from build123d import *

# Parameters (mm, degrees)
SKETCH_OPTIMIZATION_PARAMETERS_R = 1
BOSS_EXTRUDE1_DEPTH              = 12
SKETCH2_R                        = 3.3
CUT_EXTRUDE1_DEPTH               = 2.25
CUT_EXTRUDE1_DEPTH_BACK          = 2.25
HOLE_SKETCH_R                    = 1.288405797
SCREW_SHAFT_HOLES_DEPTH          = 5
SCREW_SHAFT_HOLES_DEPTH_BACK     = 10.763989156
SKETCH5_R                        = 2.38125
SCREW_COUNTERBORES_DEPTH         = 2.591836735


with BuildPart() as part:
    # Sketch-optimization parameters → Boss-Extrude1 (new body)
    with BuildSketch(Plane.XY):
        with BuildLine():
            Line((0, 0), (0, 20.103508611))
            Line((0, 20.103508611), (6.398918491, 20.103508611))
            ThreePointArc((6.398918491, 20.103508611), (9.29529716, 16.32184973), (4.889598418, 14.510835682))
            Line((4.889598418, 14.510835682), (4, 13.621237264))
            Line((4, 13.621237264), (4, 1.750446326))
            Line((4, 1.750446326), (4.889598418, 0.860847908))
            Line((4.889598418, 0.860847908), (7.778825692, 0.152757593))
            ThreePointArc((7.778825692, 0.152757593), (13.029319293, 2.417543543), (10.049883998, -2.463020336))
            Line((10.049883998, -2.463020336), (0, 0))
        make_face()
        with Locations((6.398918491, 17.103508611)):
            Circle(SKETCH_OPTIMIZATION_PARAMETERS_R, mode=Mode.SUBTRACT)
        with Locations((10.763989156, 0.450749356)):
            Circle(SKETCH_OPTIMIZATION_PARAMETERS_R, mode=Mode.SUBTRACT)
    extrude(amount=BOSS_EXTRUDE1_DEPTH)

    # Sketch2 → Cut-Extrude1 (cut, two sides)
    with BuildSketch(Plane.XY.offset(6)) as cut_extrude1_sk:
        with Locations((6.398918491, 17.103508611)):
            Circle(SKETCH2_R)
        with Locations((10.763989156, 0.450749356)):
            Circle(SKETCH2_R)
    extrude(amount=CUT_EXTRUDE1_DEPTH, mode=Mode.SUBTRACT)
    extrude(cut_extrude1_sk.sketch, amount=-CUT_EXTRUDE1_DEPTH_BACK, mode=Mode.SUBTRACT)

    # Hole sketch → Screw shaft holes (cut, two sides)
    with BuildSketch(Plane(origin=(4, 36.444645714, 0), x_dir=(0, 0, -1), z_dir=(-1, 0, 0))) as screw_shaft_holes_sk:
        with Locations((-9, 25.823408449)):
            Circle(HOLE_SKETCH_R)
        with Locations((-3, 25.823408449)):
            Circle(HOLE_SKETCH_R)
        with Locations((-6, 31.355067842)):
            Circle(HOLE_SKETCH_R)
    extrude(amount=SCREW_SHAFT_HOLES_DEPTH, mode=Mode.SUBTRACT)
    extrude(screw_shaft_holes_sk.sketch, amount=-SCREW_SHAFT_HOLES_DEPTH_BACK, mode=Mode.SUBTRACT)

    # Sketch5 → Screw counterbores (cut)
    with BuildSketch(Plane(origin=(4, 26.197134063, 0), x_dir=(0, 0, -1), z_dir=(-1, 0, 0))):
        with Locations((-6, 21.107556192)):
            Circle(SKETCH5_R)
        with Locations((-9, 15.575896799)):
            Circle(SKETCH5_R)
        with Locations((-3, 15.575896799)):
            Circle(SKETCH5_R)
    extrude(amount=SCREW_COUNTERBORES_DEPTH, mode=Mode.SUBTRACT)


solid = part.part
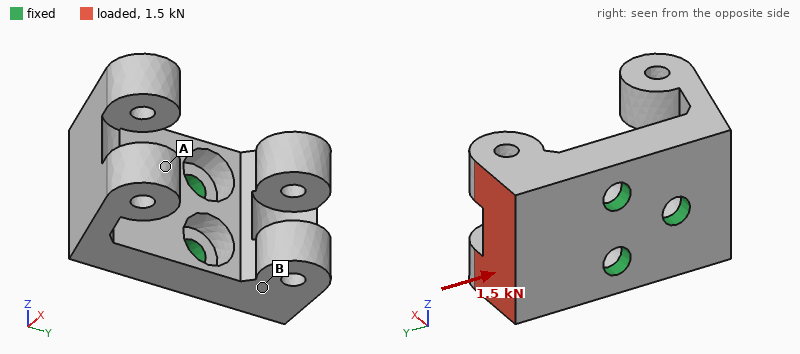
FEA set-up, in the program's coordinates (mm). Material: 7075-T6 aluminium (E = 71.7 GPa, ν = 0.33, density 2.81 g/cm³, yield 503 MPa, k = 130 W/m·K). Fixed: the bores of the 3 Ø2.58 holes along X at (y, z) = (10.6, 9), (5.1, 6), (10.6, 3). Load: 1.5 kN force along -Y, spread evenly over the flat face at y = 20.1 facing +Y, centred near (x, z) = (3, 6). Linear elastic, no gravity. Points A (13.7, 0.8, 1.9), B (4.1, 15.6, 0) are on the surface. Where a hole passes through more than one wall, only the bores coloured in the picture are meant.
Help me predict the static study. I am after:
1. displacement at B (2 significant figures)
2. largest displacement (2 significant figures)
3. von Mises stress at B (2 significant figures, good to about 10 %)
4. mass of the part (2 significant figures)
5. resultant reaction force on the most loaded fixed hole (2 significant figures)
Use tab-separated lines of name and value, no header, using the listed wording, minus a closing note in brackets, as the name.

displacement at B	32 µm
largest displacement	72 µm
von Mises stress at B	54 MPa
mass of the part	3.7 g
resultant reaction force on the most loaded fixed hole	590 N
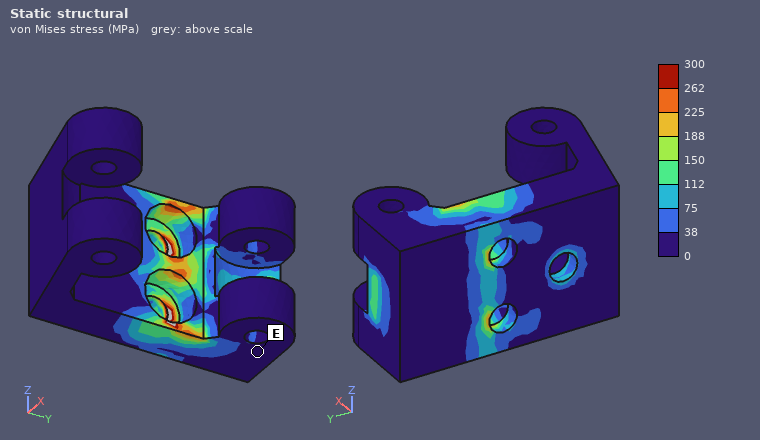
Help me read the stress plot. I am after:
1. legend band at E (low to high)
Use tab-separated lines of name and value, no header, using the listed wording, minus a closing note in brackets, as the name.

legend band at E	0 to 38 MPa
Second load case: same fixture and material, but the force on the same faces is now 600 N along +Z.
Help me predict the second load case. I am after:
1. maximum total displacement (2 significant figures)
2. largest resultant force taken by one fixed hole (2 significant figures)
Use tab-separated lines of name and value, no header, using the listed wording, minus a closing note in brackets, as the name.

maximum total displacement	21 µm
largest resultant force taken by one fixed hole	730 N
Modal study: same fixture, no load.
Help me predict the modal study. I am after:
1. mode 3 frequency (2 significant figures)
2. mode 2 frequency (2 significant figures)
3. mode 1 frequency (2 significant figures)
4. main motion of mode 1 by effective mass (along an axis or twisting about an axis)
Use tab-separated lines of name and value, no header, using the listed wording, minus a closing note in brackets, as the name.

mode 3 frequency	13 kHz
mode 2 frequency	11 kHz
mode 1 frequency	9600 Hz
main motion of mode 1 by effective mass	along Y
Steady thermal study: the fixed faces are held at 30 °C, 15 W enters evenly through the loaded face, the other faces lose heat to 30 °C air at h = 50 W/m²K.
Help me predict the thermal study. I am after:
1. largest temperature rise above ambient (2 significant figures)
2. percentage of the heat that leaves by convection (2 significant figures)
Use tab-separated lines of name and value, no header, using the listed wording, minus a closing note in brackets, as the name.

largest temperature rise above ambient	30 K
percentage of the heat that leaves by convection	3.3 %
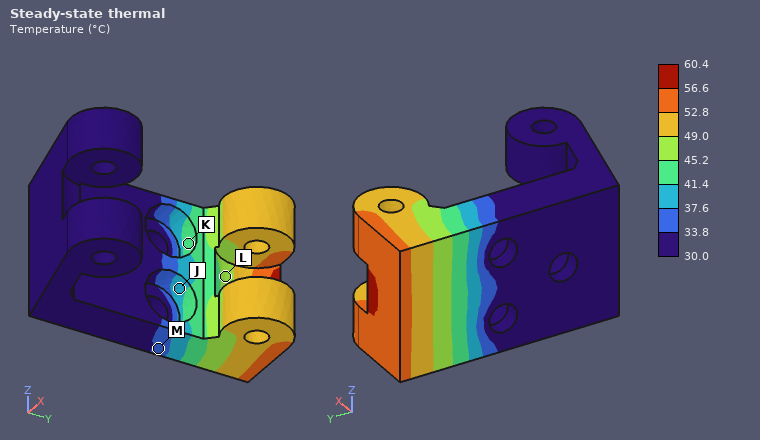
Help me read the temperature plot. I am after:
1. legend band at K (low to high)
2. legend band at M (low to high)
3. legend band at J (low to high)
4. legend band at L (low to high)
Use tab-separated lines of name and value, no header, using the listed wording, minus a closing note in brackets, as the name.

legend band at K	41.4 to 45.2 °C
legend band at M	33.8 to 37.6 °C
legend band at J	37.6 to 41.4 °C
legend band at L	45.2 to 49.0 °C
